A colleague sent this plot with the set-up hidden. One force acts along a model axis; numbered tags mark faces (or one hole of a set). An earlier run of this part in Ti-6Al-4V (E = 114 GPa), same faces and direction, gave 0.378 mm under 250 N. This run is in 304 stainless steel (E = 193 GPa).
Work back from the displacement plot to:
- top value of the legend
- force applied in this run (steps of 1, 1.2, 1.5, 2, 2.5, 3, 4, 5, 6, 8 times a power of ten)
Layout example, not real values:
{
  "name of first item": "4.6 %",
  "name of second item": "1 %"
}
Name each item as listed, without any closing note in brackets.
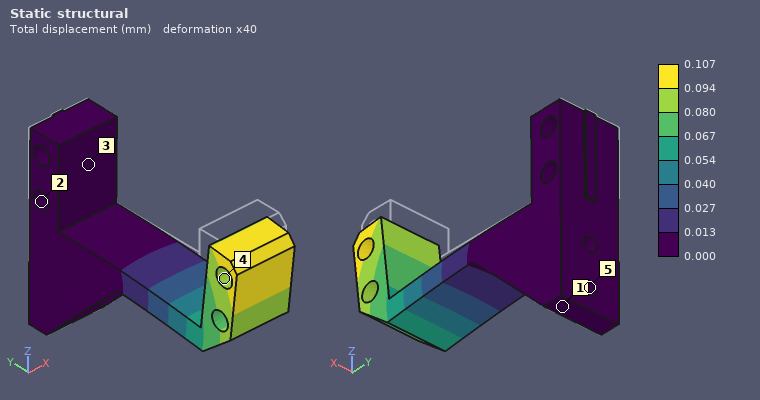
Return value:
{
  "top value of the legend": "0.107 mm",
  "force applied in this run": "120 N"
}
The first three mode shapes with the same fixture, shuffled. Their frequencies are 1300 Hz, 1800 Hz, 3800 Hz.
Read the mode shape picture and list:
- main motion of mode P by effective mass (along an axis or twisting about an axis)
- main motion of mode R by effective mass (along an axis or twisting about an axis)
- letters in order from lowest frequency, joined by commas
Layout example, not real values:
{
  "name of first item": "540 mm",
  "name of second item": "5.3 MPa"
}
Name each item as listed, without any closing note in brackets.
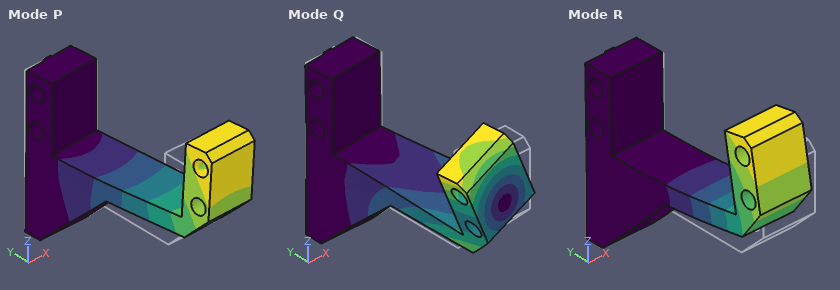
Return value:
{
  "main motion of mode P by effective mass": "along X",
  "main motion of mode R by effective mass": "along Z",
  "letters in order from lowest frequency, joined by commas": "R, P, Q"
}
